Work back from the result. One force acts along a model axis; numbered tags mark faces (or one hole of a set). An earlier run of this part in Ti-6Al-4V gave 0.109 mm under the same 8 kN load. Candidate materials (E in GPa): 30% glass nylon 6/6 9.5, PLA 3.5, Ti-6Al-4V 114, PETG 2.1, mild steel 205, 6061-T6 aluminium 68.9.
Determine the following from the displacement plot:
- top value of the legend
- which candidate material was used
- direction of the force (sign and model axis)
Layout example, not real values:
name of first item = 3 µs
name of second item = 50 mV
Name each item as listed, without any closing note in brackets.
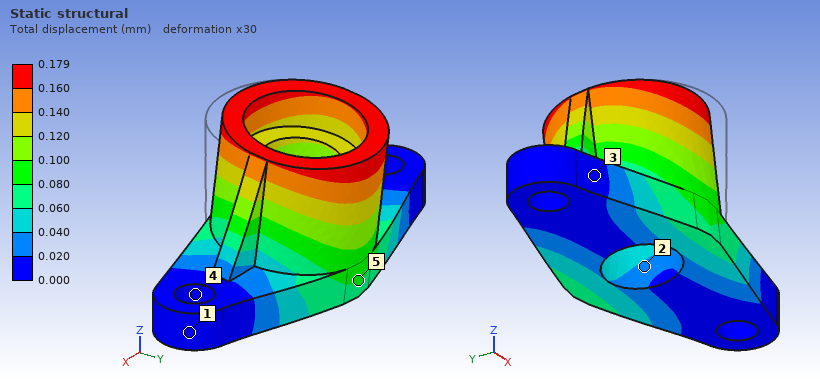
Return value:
top value of the legend = 0.179 mm
which candidate material was used = 6061-T6 aluminium
direction of the force = +Y
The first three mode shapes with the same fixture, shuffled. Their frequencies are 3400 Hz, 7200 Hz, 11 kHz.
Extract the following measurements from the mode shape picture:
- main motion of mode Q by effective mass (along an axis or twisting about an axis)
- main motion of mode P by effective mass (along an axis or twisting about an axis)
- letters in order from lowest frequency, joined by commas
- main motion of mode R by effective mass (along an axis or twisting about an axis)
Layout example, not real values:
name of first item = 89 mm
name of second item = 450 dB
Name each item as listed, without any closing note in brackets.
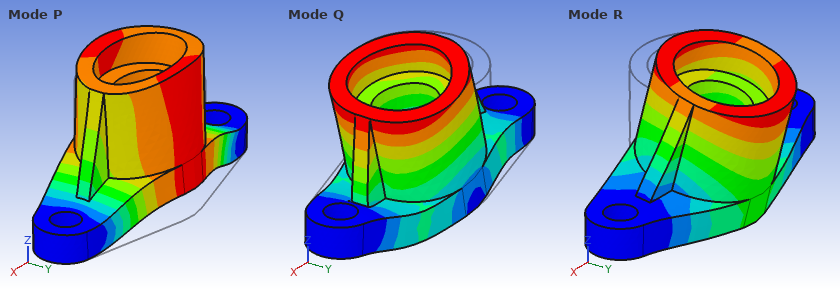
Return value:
main motion of mode Q by effective mass = along X
main motion of mode P by effective mass = along Z
letters in order from lowest frequency, joined by commas = R, P, Q
main motion of mode R by effective mass = along Y
